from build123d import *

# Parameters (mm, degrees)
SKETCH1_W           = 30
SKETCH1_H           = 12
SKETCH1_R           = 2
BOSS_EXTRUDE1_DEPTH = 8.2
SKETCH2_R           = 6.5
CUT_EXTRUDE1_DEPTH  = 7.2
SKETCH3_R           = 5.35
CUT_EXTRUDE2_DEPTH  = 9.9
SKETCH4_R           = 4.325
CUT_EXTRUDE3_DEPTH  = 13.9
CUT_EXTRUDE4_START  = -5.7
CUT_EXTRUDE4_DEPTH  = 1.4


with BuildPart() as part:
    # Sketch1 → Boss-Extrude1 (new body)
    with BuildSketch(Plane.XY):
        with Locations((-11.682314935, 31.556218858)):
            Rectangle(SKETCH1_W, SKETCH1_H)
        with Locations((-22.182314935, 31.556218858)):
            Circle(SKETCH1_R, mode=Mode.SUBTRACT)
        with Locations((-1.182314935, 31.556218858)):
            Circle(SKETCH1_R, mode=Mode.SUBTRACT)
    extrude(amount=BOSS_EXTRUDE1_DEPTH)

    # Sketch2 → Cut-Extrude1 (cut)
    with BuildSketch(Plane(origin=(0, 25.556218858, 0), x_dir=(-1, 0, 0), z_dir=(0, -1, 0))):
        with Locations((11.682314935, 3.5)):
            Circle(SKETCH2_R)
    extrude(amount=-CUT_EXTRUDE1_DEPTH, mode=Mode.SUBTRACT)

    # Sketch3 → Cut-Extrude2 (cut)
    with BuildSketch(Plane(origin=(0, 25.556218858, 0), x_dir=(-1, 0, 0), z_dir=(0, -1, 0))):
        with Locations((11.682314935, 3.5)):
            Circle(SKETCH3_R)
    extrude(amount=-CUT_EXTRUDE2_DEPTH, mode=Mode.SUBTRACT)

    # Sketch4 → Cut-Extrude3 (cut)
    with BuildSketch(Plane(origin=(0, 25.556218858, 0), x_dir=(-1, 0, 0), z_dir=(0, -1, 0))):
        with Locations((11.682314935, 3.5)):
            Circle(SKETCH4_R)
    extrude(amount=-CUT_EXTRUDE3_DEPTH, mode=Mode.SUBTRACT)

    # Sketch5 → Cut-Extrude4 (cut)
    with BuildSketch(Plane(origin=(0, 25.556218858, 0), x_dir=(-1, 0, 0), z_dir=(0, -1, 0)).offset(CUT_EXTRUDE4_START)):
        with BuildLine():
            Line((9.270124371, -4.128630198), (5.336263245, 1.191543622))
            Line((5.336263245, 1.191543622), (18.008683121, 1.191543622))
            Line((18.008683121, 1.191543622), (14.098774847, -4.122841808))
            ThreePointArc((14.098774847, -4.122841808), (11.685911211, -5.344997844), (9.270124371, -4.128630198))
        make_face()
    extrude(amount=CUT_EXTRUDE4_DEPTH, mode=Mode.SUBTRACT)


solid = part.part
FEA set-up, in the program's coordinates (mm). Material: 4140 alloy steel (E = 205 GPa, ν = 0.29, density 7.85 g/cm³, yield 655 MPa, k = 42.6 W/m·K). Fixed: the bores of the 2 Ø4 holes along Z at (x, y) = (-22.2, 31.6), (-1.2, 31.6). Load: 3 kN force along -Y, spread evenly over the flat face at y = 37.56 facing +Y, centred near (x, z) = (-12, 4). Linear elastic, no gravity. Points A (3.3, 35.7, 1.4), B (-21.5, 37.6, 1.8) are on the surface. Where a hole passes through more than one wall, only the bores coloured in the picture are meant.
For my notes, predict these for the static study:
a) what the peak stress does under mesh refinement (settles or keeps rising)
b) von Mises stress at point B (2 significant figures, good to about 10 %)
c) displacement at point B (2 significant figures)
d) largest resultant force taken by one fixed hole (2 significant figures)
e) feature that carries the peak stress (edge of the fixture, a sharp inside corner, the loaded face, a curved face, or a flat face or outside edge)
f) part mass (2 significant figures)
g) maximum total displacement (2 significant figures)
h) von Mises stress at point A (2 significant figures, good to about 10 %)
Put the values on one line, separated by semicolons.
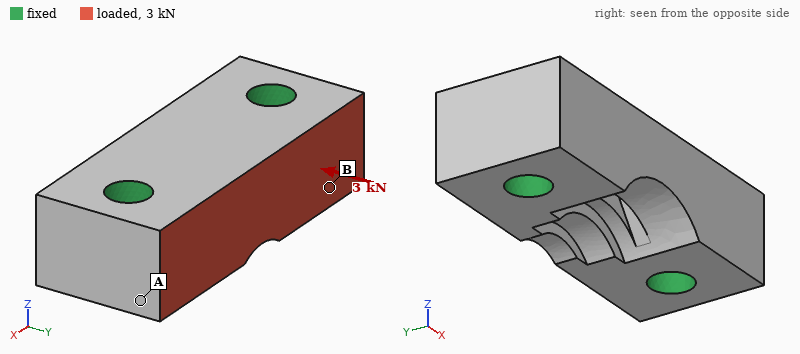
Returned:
keeps rising; 20 MPa; 0.44 µm; 1.5 kN; edge of the fixture; 20 g; 1.6 µm; 10 MPa
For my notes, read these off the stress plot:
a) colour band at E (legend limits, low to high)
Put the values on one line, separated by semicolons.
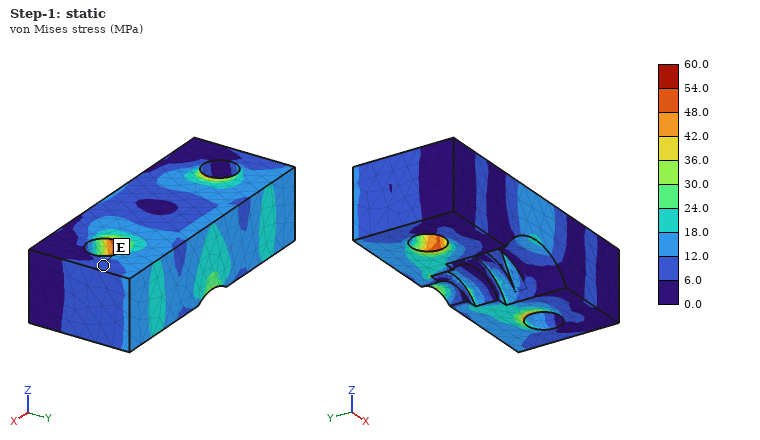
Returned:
6.0 to 12.0 MPa
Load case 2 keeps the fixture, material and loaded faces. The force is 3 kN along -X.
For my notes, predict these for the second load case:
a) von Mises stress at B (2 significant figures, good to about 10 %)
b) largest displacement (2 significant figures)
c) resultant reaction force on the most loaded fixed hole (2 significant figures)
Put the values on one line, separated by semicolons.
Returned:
23 MPa; 1.9 µm; 1.6 kN
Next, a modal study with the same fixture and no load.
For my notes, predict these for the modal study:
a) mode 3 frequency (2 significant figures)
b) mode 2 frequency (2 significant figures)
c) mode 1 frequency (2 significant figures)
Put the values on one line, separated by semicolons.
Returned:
75 kHz; 63 kHz; 62 kHz
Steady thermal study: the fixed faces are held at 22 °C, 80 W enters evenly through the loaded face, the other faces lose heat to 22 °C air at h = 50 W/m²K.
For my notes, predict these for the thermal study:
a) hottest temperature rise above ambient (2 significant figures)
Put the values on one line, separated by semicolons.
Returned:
72 K
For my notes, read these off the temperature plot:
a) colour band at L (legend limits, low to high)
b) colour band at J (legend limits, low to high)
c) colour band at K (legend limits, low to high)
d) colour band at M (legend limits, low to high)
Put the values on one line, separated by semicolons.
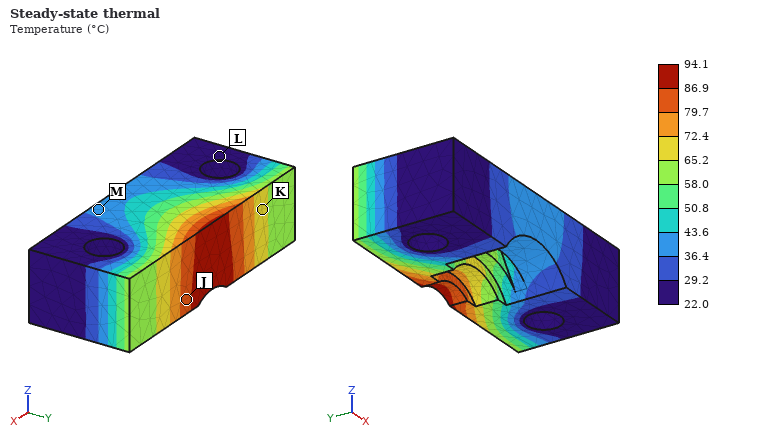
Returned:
22.0 to 29.2 °C; 79.7 to 86.9 °C; 65.2 to 72.4 °C; 36.4 to 43.6 °C
